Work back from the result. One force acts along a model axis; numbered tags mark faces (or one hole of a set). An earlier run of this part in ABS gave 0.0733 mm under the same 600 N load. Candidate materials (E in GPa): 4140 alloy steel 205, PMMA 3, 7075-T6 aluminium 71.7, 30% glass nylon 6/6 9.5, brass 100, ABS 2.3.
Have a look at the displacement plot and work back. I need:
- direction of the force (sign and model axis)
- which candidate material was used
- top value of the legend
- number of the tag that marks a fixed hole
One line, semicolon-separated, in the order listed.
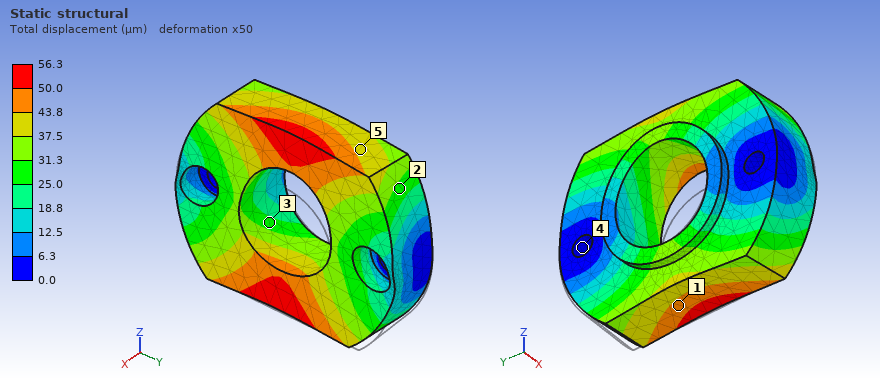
+Z; PMMA; 56.3 µm; 4
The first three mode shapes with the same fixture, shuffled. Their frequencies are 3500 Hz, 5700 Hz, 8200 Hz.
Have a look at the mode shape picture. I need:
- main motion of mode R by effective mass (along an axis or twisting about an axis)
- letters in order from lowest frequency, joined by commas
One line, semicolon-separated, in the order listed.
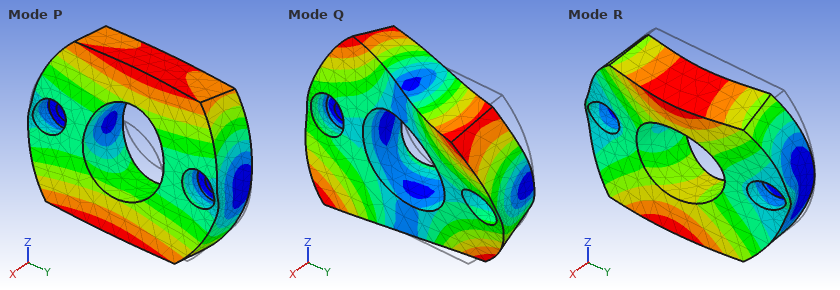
along X; P, R, Q
